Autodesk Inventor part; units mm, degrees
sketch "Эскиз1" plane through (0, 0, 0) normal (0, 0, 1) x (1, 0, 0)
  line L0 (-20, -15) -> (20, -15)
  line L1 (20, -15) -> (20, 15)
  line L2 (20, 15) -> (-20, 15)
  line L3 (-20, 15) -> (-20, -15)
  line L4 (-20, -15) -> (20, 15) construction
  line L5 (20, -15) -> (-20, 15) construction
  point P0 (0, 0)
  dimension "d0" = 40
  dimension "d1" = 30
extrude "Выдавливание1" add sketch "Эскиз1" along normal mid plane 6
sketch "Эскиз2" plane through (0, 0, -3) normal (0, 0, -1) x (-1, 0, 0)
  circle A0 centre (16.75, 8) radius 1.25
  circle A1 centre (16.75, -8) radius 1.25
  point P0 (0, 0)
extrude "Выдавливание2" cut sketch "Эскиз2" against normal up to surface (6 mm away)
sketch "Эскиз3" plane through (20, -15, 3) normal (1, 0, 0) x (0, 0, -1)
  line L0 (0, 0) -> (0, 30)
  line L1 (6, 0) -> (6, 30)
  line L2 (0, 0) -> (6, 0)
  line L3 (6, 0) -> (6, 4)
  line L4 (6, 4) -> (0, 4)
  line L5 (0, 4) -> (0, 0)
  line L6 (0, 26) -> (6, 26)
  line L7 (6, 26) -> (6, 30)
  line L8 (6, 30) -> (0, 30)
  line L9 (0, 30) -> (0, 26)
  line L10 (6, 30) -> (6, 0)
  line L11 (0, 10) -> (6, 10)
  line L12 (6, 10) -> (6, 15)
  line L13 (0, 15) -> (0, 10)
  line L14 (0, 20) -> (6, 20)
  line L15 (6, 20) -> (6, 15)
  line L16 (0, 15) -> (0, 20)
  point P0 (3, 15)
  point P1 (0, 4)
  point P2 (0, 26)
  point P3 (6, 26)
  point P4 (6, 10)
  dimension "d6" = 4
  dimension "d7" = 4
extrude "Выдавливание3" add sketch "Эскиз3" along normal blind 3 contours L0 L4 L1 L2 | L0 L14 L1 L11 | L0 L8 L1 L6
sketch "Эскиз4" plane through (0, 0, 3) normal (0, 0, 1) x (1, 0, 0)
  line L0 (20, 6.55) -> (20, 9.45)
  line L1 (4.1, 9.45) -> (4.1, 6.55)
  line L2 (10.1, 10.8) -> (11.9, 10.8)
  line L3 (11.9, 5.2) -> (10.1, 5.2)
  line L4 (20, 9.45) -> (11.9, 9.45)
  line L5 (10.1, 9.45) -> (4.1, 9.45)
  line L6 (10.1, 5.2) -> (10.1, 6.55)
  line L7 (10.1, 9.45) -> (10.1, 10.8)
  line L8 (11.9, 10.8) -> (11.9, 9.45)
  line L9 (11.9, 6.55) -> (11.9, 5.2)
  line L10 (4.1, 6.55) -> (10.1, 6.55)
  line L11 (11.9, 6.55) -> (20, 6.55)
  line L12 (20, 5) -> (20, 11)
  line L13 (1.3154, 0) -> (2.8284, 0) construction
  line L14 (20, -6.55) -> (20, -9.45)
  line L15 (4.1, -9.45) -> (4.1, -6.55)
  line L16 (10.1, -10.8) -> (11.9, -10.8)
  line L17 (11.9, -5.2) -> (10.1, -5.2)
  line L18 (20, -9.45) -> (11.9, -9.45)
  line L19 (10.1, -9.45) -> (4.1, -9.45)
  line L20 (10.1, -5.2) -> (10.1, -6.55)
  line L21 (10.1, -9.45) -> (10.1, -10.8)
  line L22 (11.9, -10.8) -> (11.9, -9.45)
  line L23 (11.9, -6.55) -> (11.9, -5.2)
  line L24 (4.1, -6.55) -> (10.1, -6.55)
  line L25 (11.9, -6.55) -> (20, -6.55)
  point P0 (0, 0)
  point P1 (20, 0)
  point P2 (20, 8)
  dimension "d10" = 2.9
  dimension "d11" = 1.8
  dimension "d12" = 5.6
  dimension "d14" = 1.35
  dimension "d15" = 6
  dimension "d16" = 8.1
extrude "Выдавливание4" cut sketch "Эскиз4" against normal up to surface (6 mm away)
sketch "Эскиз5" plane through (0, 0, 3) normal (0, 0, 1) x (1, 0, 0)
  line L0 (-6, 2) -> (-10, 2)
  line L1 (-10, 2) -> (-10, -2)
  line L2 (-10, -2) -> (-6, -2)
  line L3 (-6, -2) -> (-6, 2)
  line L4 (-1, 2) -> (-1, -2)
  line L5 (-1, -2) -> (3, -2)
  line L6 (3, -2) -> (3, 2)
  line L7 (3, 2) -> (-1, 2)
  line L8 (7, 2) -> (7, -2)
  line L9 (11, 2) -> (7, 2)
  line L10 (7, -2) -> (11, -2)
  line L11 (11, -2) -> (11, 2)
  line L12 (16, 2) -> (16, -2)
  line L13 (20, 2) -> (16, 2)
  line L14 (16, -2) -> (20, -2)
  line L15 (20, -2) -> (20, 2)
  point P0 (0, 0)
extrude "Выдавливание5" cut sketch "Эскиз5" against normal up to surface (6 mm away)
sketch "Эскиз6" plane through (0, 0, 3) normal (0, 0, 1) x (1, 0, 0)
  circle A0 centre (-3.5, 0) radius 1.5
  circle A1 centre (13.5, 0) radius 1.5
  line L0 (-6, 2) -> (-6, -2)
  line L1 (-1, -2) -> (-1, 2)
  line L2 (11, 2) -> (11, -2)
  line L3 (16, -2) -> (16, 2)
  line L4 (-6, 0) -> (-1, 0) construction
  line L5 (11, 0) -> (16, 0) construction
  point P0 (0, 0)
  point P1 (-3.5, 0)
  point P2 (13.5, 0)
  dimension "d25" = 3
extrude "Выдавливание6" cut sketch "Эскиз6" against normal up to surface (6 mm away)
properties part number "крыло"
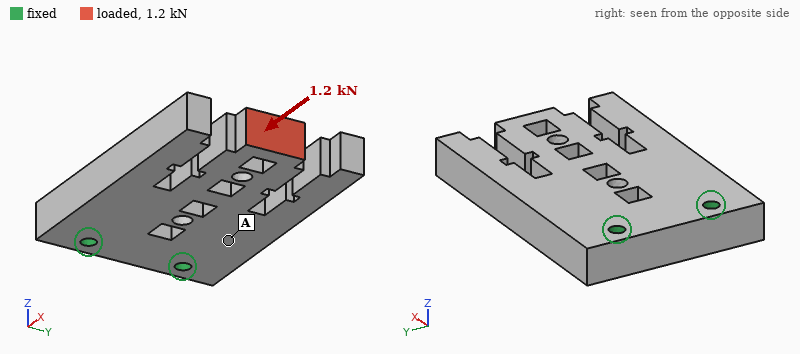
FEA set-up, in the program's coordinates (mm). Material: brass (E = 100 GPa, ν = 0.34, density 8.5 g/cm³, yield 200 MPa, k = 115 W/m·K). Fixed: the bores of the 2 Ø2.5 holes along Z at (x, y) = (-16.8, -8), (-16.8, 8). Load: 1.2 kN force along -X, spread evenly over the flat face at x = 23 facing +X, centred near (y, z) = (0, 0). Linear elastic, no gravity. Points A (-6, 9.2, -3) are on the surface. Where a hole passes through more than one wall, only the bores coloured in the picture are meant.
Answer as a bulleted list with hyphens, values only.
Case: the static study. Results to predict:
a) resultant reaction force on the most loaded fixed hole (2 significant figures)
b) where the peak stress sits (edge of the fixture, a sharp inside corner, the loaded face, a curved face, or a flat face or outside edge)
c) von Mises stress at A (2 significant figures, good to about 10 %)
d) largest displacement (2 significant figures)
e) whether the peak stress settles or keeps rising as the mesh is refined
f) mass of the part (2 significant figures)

- 610 N
- a sharp inside corner
- 8.2 MPa
- 8.8 µm
- keeps rising
- 54 g
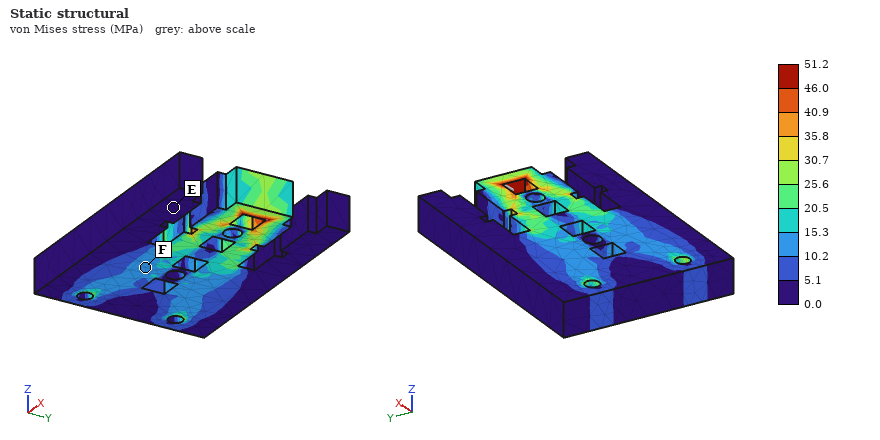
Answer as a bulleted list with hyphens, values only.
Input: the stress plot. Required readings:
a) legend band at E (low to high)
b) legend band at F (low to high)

- 0.0 to 5.1 MPa
- 10.2 to 15.3 MPa
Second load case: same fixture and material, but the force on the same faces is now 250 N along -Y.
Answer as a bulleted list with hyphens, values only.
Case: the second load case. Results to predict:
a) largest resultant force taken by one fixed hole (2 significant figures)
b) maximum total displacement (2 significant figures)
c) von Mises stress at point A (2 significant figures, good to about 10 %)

- 570 N
- 25 µm
- 8.0 MPa
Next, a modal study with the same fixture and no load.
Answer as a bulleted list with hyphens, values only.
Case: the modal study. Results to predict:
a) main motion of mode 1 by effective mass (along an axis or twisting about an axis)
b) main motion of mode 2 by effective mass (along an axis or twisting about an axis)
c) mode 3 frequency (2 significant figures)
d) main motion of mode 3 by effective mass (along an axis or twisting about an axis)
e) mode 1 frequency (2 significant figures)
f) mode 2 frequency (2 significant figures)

- along Z
- twisting about X
- 5000 Hz
- along Y
- 2200 Hz
- 4000 Hz
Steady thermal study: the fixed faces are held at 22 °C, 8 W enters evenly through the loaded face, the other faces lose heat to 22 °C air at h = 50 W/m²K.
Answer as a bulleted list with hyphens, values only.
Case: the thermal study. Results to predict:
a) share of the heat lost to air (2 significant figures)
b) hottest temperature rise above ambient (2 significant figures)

- 20 %
- 35 K
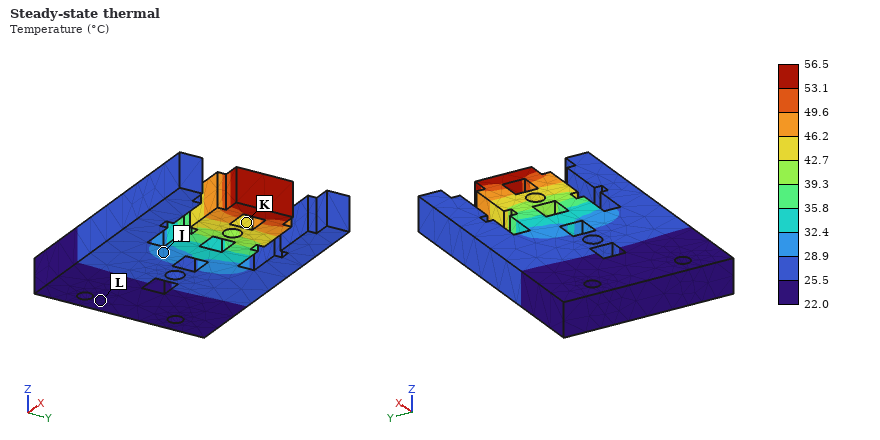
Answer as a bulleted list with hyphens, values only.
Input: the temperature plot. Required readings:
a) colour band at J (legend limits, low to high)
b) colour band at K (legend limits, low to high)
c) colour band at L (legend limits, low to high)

- 28.9 to 32.4 °C
- 42.7 to 46.2 °C
- 22.0 to 25.5 °C
